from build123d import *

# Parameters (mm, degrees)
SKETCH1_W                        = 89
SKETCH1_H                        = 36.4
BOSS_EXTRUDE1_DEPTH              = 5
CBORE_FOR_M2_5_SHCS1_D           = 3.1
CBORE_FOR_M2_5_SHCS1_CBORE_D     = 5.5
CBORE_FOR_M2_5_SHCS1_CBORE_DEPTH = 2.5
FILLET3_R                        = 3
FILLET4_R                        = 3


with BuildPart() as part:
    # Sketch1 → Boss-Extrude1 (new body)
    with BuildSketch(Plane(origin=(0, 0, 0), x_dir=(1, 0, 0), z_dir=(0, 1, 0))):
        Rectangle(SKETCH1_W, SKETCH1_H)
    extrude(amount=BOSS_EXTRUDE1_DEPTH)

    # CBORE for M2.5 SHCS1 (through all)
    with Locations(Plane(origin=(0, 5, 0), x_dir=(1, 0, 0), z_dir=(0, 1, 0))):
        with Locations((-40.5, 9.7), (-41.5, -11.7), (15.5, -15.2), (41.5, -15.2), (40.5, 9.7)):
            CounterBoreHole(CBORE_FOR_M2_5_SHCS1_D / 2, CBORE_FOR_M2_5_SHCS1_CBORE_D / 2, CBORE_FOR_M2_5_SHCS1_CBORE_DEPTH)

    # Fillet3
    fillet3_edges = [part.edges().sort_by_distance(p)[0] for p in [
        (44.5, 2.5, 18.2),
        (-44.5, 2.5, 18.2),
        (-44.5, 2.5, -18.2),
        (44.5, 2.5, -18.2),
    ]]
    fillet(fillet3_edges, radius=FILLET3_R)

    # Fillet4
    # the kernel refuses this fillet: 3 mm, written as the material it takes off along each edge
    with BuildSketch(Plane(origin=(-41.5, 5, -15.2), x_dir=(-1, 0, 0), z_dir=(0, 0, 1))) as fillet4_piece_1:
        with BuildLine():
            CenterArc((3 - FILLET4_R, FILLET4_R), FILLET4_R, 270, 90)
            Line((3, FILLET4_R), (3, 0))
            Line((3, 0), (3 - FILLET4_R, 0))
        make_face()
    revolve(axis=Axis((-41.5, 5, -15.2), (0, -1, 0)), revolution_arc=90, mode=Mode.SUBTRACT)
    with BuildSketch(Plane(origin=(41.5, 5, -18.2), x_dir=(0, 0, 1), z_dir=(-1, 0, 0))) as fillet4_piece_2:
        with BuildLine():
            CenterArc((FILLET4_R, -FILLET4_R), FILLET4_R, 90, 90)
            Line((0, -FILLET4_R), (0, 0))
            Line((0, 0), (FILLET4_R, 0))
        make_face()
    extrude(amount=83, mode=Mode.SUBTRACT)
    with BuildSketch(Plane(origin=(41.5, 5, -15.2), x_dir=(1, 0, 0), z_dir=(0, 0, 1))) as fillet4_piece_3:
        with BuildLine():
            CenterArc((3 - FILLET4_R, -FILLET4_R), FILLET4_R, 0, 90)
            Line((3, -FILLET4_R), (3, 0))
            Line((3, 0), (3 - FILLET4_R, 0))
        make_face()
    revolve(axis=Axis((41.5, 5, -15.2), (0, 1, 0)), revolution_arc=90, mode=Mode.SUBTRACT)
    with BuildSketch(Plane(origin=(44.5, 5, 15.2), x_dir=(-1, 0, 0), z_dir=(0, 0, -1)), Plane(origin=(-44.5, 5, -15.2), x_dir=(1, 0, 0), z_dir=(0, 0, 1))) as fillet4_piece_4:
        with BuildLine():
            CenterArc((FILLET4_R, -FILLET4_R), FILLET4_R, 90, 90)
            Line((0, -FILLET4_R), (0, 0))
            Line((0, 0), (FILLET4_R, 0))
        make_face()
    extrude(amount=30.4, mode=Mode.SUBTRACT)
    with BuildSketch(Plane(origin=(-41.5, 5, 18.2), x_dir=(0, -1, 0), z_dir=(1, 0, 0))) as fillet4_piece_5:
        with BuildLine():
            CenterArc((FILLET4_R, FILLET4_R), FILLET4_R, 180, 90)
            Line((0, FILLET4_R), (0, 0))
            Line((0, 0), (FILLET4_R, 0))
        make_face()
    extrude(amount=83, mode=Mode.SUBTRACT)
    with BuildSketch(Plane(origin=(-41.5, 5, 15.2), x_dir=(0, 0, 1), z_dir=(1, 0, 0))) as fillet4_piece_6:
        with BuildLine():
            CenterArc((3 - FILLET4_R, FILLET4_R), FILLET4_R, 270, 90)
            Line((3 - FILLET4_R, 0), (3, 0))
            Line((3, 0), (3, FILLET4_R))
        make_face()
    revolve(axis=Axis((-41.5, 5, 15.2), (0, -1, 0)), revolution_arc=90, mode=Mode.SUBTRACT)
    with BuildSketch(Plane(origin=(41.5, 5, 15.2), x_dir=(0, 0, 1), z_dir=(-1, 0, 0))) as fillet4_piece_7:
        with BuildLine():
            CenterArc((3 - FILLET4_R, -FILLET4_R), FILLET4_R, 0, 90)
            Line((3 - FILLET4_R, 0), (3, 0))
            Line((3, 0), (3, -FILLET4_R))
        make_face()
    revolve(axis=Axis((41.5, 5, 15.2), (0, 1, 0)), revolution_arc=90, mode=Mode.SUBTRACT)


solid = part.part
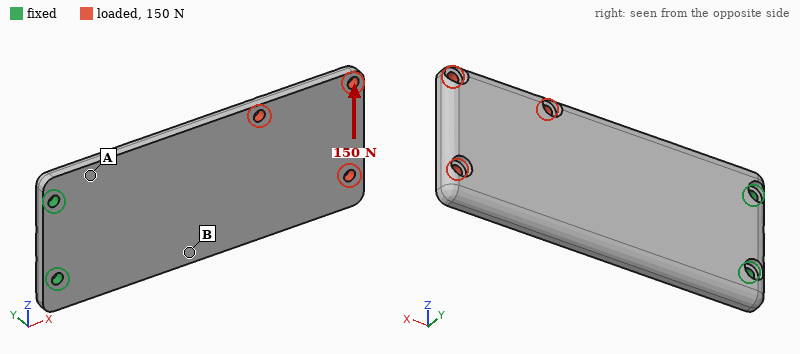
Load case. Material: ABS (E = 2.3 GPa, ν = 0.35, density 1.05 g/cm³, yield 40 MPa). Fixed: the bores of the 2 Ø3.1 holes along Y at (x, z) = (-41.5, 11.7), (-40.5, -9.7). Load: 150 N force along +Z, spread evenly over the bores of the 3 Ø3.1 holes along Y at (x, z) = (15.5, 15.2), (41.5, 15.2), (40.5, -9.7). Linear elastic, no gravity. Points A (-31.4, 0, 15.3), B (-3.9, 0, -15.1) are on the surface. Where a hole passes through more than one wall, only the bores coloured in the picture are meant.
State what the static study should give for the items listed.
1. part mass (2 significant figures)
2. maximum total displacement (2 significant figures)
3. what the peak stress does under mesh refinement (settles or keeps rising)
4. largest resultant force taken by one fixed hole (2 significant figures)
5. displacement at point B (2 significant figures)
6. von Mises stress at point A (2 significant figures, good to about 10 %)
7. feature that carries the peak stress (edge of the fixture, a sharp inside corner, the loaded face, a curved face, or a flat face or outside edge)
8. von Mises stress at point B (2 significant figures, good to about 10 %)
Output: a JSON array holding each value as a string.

["16 g", "1.1 mm", "keeps rising", "490 N", "0.44 mm", "10 MPa", "edge of the fixture", "4.8 MPa"]
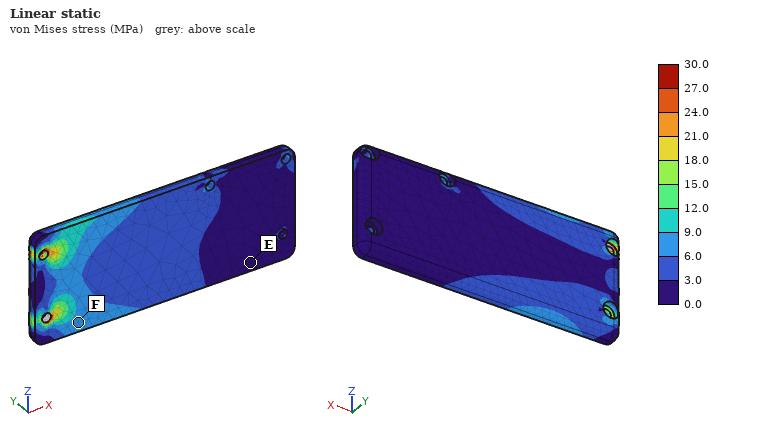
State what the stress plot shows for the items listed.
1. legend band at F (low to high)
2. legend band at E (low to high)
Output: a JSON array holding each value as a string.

["6.0 to 9.0 MPa", "0.0 to 3.0 MPa"]
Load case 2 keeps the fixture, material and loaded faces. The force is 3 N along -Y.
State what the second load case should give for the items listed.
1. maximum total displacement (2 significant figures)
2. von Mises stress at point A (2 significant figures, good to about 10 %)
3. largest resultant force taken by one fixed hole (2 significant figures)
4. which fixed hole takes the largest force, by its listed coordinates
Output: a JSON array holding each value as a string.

["0.88 mm", "1.3 MPa", "1.8 N", "(-41.5, 11.7)"]
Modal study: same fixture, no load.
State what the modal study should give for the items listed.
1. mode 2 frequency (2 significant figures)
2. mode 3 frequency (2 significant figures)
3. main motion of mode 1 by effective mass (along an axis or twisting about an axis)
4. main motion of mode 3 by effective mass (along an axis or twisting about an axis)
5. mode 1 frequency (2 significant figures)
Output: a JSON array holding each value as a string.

["740 Hz", "870 Hz", "along Y", "along Z", "130 Hz"]
